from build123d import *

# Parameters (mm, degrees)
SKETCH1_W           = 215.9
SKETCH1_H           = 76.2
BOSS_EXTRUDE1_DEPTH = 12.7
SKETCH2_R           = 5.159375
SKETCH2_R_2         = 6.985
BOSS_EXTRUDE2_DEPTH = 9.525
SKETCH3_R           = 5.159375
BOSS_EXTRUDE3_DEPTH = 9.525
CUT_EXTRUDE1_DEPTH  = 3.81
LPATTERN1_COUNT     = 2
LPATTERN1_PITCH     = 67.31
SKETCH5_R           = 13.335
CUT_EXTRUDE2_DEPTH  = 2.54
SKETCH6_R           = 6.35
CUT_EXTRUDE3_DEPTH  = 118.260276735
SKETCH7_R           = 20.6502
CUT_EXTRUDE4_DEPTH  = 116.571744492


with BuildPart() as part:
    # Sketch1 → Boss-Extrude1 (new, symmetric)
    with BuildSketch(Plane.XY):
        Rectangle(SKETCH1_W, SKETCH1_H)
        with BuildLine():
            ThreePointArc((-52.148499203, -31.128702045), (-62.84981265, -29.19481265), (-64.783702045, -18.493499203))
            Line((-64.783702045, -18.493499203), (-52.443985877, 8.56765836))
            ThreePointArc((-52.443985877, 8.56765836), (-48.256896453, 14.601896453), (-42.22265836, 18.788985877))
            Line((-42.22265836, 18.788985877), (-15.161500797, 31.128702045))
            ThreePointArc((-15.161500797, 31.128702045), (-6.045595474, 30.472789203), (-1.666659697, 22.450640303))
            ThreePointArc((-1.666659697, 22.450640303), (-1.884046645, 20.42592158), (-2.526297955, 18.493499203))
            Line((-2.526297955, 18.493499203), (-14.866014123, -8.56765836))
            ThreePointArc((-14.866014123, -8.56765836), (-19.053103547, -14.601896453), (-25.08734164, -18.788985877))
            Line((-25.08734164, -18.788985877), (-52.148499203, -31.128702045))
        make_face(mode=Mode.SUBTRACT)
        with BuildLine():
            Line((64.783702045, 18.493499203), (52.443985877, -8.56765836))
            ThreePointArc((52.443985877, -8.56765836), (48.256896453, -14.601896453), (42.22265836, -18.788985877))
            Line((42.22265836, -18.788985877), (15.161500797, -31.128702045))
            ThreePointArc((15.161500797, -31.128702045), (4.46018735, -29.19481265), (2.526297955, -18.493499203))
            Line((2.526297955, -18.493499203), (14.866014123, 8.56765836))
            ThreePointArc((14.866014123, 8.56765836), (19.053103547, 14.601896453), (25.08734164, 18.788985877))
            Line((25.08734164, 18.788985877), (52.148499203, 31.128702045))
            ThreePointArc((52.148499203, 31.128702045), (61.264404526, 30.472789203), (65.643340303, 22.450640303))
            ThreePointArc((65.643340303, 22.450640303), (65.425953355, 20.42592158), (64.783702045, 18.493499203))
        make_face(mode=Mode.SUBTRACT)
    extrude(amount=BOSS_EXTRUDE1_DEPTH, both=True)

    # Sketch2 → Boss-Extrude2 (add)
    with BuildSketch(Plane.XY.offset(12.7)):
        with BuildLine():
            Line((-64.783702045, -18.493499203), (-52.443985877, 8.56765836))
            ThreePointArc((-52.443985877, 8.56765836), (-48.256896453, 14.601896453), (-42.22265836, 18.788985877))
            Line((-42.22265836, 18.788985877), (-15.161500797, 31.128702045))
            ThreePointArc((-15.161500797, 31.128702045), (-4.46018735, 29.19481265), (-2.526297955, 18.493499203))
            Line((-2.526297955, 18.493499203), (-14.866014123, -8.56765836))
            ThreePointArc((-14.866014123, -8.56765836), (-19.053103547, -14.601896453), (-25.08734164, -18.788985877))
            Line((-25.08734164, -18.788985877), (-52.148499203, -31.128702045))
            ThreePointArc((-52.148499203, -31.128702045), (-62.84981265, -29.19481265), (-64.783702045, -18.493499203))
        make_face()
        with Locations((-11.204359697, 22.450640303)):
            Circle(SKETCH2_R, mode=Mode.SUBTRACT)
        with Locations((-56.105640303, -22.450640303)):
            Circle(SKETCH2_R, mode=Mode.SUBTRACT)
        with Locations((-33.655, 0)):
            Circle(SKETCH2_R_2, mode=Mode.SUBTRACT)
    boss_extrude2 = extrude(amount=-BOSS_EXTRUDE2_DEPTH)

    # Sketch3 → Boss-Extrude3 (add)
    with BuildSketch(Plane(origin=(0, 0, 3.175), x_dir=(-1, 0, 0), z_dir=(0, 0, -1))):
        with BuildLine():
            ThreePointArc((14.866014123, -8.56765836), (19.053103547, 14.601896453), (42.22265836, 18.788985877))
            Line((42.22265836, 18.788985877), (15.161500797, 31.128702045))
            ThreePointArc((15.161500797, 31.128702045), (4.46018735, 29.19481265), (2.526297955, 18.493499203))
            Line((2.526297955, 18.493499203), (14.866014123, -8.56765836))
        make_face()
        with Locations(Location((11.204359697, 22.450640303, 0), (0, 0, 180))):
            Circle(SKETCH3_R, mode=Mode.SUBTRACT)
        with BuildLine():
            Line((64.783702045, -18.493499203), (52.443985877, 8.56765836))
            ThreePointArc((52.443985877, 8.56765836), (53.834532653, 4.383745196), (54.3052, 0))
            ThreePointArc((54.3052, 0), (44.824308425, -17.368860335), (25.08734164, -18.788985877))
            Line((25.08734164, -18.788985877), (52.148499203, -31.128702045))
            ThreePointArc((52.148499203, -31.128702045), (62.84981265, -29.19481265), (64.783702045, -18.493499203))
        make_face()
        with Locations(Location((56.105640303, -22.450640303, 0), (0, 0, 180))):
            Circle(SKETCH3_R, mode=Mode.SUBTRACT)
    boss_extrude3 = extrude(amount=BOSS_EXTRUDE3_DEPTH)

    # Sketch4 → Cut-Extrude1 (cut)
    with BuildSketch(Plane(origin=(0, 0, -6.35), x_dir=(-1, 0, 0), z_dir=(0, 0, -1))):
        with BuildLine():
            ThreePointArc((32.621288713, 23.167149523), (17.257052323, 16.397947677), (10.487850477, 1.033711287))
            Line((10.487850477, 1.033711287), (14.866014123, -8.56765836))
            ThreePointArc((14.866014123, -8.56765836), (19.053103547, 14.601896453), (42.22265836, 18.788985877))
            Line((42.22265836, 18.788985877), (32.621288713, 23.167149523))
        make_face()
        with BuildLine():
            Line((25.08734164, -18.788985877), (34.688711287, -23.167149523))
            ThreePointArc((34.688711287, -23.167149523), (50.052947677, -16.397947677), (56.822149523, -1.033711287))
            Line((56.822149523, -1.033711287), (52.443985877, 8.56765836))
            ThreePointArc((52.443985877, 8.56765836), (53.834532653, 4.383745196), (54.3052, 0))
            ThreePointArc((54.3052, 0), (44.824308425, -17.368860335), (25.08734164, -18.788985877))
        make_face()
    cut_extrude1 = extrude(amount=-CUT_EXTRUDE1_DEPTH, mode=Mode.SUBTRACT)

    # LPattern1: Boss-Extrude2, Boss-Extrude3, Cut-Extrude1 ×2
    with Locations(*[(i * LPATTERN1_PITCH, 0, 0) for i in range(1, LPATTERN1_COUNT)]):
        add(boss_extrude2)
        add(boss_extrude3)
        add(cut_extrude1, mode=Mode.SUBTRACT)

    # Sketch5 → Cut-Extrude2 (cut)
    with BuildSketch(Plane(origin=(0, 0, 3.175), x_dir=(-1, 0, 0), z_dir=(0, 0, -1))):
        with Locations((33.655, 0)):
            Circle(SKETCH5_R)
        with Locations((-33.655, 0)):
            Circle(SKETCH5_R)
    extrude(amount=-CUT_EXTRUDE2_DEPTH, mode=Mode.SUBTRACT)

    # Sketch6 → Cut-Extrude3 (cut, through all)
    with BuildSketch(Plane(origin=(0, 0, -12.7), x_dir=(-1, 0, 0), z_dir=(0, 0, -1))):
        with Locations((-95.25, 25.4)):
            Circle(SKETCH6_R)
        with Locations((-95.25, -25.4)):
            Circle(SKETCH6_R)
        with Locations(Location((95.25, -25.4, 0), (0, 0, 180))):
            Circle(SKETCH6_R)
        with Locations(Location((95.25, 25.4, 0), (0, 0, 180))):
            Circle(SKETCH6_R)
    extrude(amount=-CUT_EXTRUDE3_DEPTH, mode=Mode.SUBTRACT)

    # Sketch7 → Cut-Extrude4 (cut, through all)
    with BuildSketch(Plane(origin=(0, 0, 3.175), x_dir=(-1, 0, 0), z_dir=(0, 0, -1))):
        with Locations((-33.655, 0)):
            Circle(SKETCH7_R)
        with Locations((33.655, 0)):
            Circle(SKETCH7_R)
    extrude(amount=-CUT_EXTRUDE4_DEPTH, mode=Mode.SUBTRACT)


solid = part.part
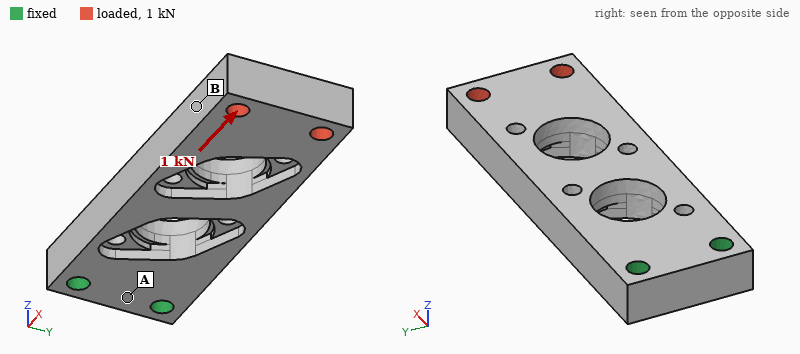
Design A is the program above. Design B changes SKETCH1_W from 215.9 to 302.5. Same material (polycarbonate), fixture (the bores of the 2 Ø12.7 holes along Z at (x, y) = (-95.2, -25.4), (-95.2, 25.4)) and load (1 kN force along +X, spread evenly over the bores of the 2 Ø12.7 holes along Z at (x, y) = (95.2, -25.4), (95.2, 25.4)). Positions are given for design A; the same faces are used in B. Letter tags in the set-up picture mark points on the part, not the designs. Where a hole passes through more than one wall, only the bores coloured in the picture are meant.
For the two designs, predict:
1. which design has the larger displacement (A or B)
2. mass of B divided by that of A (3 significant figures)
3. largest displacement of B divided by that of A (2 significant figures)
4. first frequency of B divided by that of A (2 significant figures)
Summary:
B
1.53
1.3
0.63
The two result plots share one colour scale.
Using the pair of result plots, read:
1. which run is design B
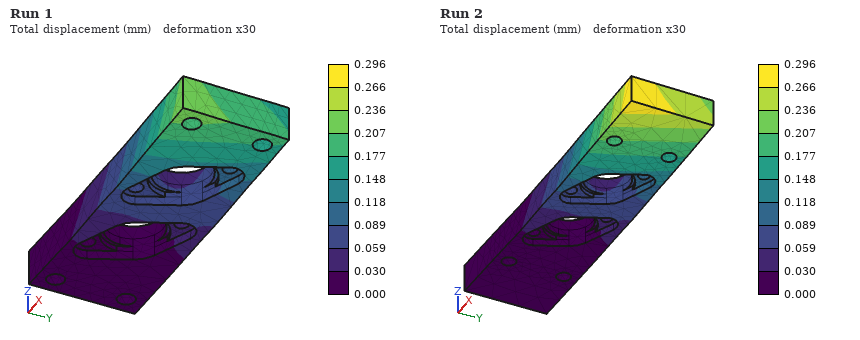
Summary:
Run 2
